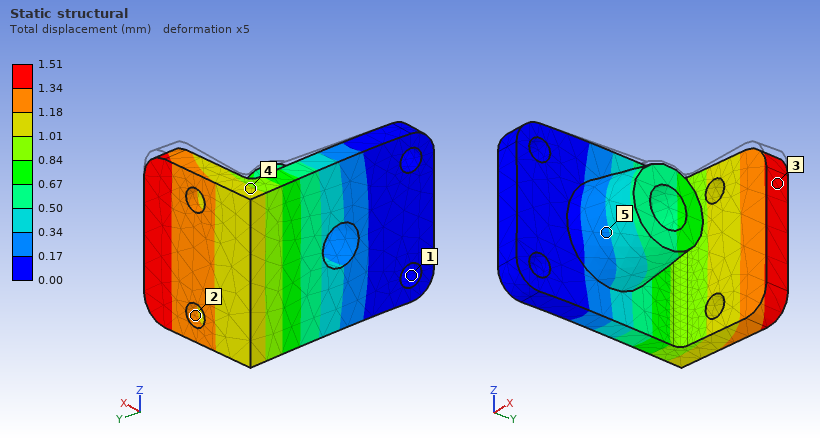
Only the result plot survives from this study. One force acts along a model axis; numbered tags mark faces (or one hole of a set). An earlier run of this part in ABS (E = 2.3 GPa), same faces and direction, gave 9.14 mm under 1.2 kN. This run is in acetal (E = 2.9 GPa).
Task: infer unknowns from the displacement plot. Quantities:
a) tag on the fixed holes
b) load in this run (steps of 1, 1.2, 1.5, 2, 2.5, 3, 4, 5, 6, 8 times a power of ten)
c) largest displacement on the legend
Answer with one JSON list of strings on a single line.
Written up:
["1", "250 N", "1.51 mm"]
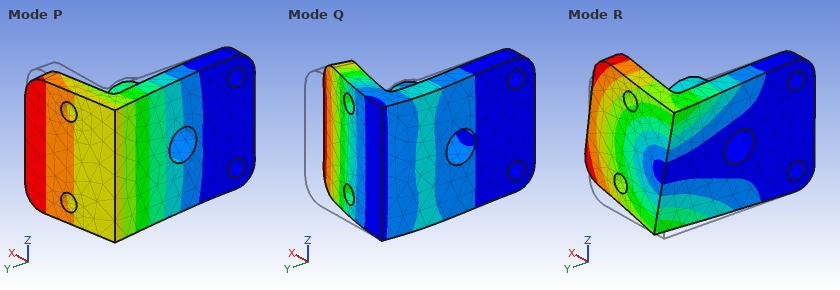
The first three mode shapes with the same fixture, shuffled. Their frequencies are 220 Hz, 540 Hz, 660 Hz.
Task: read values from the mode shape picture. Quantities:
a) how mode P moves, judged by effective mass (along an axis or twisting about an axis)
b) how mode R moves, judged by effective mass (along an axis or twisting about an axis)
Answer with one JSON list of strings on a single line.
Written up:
["along X", "along Z"]
